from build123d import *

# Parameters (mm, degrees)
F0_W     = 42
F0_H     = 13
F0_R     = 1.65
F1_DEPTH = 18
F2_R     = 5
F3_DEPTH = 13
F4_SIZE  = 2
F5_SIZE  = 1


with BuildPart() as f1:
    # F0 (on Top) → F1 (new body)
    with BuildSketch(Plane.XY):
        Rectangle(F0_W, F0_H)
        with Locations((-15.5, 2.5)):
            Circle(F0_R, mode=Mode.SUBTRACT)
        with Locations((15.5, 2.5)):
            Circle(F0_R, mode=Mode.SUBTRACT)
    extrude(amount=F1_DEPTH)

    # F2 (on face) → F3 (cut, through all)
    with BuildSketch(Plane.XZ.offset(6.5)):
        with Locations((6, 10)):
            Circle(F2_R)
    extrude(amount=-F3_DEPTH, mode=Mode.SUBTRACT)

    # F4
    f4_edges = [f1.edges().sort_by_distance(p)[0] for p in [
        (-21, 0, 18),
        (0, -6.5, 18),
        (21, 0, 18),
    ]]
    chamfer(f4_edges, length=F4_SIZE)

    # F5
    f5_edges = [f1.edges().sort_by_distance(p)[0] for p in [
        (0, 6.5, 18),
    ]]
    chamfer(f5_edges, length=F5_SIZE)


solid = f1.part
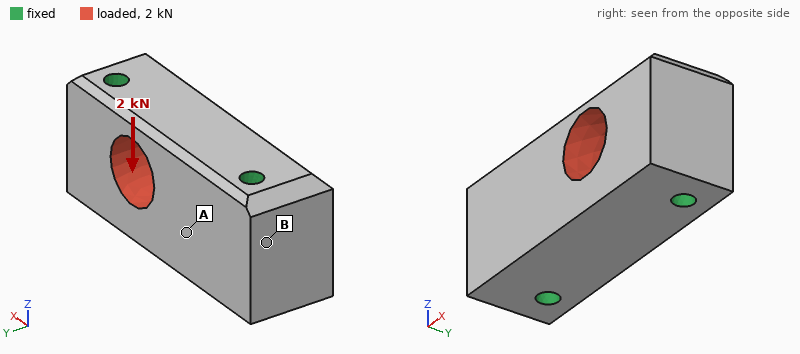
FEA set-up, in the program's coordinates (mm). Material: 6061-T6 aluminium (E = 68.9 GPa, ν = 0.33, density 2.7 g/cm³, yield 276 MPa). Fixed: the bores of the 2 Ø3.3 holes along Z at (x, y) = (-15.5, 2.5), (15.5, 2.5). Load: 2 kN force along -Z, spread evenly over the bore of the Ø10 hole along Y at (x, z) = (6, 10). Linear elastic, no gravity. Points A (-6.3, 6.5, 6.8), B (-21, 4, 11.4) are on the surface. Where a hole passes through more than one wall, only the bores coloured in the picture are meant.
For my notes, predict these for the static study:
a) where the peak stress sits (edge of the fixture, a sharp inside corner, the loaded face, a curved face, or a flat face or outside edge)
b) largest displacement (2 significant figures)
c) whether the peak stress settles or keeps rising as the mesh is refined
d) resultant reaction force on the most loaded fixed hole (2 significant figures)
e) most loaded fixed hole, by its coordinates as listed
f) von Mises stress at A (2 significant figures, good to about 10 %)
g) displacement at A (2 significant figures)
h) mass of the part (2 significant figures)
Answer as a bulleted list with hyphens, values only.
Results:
- edge of the fixture
- 5.3 µm
- keeps rising
- 1.3 kN
- (15.5, 2.5)
- 9.1 MPa
- 1.9 µm
- 23 g
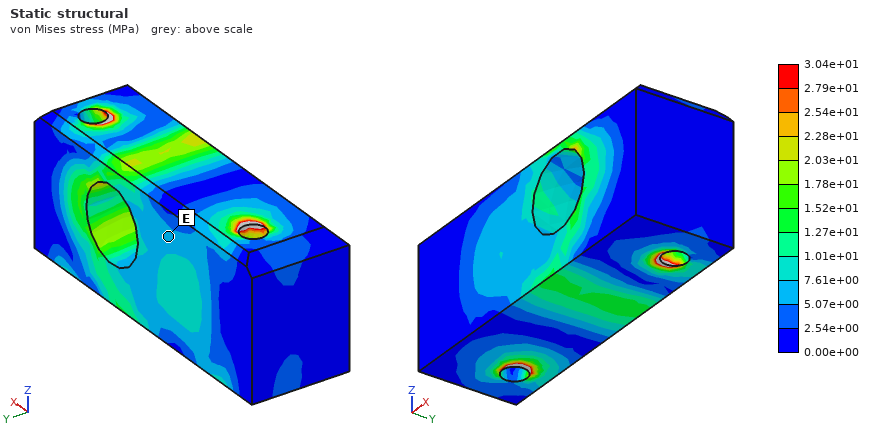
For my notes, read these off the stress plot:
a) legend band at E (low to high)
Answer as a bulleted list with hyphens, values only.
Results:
- 5.07e+00 to 7.61e+00 MPa
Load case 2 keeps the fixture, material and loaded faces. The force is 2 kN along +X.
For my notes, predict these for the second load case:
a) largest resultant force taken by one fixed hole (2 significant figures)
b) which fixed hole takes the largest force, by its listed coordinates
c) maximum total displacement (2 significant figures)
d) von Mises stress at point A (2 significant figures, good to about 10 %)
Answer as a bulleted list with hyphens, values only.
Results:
- 1.2 kN
- (15.5, 2.5)
- 1.7 µm
- 4.9 MPa
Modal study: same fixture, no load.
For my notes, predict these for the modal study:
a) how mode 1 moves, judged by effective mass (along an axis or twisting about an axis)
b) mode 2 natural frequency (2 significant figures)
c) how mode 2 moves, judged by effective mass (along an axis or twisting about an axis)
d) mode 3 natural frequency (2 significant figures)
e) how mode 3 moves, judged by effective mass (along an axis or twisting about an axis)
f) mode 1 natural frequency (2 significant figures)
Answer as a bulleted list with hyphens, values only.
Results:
- along Y
- 35 kHz
- along Z
- 42 kHz
- twisting about X
- 30 kHz
